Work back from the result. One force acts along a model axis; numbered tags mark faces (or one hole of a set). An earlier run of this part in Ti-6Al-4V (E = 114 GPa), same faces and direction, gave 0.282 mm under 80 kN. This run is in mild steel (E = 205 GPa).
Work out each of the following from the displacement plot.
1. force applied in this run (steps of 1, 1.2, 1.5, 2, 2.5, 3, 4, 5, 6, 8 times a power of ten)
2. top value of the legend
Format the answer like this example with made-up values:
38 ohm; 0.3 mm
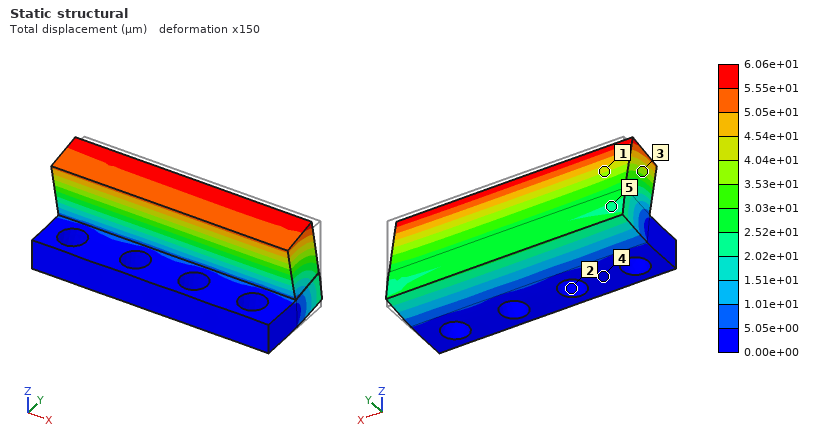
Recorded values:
30 kN; 6.06e+01 µm
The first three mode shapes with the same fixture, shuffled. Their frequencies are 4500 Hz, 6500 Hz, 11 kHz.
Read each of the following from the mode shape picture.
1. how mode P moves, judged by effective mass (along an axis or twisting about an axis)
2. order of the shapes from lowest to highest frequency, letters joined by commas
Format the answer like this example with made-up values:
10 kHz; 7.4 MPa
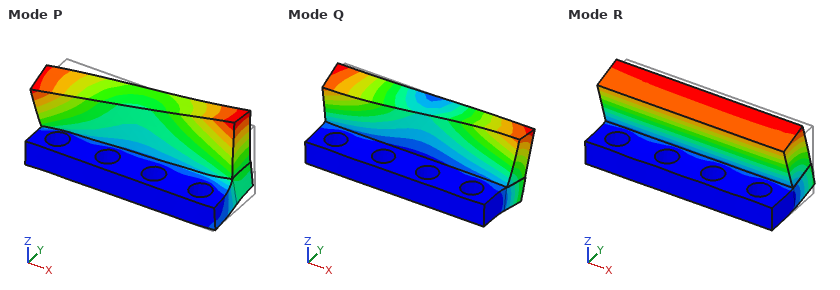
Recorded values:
along X; R, Q, P
